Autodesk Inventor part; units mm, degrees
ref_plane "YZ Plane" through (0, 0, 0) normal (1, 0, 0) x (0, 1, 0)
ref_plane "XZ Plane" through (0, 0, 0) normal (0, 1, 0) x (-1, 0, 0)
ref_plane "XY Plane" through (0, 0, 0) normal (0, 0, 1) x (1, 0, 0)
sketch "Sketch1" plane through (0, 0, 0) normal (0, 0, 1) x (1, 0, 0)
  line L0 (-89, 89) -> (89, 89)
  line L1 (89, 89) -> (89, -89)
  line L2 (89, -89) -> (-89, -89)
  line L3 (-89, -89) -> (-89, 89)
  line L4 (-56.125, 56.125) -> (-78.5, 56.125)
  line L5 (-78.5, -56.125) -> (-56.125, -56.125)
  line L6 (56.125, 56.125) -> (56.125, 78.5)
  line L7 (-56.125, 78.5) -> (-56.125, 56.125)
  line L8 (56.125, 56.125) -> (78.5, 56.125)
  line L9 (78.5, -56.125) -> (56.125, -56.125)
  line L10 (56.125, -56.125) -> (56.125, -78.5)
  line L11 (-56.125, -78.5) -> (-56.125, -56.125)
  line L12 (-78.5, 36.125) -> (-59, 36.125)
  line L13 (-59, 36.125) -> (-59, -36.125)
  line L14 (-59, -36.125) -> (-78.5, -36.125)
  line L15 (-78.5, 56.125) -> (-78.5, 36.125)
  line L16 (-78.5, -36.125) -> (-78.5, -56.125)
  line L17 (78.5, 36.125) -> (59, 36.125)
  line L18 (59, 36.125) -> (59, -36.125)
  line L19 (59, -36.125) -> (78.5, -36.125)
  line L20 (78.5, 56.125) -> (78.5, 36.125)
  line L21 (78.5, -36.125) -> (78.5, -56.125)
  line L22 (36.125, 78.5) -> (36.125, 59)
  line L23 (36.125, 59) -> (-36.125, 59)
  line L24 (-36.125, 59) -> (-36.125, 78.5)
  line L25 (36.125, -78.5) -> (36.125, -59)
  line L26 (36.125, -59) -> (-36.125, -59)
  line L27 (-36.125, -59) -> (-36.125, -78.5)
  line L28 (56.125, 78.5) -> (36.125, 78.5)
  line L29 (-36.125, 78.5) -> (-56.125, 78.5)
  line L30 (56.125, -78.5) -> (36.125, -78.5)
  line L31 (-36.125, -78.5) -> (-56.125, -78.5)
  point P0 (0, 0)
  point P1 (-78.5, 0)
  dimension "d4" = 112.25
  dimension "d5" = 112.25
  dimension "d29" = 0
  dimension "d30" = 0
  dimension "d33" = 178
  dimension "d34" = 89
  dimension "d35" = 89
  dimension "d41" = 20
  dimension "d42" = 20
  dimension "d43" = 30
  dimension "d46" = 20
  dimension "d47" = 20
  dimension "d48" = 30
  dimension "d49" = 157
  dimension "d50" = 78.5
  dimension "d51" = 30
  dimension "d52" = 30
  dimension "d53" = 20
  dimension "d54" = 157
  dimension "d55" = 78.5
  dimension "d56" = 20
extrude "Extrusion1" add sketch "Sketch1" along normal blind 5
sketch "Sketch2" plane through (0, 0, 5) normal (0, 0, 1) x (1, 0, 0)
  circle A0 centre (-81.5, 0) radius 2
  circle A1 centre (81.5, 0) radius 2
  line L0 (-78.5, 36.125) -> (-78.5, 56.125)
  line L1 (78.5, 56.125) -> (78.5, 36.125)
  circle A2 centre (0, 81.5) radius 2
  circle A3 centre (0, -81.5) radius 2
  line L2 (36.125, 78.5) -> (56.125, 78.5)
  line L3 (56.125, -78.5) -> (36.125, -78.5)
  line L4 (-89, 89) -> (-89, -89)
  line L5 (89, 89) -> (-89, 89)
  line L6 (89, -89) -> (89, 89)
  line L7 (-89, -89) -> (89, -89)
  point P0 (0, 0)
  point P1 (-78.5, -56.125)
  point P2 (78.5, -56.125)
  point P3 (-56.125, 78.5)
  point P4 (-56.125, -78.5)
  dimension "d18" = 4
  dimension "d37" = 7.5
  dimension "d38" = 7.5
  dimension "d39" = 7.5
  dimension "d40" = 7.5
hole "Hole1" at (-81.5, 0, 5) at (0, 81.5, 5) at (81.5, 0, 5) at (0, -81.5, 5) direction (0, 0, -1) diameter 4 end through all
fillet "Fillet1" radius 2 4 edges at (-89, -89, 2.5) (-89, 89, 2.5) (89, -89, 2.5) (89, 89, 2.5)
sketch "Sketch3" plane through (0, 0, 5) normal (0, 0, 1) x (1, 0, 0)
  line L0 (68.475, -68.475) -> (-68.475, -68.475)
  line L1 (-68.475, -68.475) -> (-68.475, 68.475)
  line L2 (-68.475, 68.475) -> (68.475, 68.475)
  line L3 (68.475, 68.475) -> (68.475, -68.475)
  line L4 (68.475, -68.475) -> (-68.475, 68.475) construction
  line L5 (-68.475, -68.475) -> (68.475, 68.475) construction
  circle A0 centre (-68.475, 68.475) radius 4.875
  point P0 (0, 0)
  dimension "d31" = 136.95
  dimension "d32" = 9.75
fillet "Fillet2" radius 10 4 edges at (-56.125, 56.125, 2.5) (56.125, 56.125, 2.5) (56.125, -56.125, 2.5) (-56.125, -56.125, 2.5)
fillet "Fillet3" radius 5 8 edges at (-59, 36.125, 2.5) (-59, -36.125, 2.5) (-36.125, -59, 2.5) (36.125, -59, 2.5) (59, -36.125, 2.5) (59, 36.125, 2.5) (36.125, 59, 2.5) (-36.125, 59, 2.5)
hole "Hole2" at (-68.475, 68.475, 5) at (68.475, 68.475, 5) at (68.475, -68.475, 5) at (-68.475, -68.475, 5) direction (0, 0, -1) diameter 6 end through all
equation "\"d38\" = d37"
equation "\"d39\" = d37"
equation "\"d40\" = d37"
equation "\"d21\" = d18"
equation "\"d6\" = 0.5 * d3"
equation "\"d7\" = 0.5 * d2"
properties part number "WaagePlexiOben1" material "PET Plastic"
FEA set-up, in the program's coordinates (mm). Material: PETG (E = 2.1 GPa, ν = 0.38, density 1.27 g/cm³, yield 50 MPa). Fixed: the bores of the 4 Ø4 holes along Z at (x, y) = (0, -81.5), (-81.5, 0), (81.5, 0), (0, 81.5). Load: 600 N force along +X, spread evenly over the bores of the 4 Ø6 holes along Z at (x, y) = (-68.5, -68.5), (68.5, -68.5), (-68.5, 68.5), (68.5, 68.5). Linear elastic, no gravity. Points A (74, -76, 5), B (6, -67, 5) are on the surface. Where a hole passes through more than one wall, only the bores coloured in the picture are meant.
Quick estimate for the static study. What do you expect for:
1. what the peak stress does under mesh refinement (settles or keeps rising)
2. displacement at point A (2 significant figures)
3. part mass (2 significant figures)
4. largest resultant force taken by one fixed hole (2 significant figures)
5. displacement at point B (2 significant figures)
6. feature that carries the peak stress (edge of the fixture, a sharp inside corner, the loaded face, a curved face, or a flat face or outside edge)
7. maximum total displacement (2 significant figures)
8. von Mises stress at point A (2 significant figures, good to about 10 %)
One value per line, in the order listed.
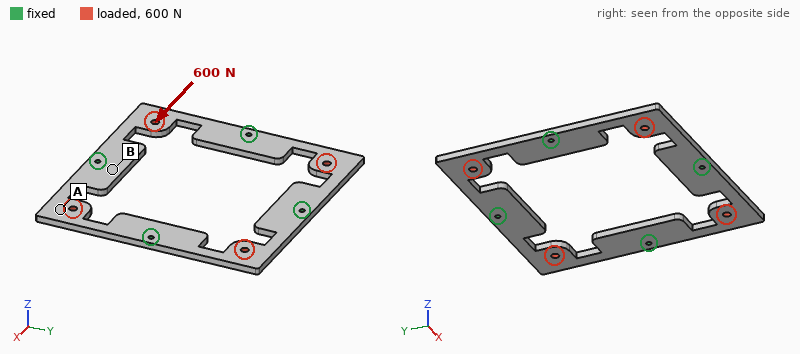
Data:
keeps rising
0.10 mm
91 g
210 N
0.031 mm
edge of the fixture
0.19 mm
1.3 MPa
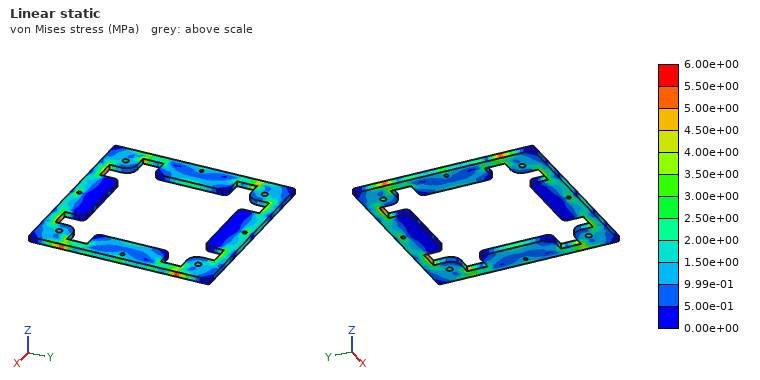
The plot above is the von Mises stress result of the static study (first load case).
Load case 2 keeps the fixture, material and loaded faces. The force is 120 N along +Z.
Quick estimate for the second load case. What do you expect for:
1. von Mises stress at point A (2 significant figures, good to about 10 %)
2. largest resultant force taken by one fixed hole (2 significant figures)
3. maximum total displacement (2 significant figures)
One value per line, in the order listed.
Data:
3.2 MPa
30 N
2.4 mm
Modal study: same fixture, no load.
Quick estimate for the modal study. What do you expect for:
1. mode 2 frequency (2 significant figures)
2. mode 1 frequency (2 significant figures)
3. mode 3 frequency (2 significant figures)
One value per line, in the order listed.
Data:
210 Hz
210 Hz
210 Hz
